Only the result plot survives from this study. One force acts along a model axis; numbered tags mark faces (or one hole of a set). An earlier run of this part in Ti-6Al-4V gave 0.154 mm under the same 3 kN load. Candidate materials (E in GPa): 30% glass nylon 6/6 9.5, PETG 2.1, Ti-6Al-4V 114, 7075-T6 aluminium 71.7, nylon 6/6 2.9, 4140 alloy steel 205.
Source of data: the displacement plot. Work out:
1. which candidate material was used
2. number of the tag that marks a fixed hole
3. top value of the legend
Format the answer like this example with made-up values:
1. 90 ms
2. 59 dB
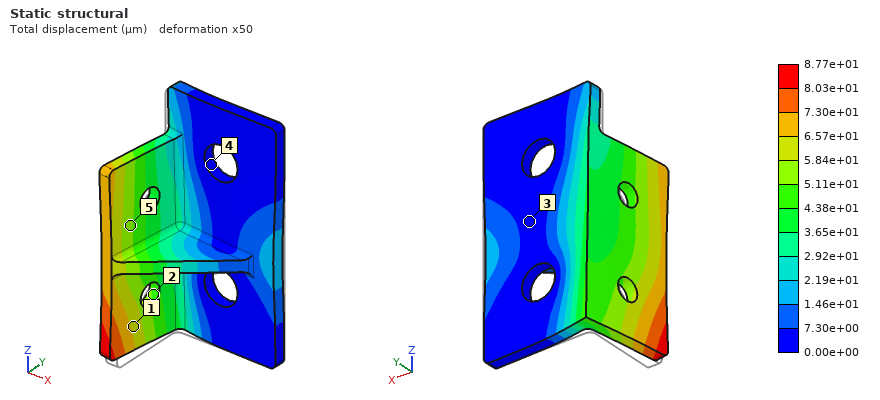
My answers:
1. 4140 alloy steel
2. 4
3. 8.77e+01 µm
